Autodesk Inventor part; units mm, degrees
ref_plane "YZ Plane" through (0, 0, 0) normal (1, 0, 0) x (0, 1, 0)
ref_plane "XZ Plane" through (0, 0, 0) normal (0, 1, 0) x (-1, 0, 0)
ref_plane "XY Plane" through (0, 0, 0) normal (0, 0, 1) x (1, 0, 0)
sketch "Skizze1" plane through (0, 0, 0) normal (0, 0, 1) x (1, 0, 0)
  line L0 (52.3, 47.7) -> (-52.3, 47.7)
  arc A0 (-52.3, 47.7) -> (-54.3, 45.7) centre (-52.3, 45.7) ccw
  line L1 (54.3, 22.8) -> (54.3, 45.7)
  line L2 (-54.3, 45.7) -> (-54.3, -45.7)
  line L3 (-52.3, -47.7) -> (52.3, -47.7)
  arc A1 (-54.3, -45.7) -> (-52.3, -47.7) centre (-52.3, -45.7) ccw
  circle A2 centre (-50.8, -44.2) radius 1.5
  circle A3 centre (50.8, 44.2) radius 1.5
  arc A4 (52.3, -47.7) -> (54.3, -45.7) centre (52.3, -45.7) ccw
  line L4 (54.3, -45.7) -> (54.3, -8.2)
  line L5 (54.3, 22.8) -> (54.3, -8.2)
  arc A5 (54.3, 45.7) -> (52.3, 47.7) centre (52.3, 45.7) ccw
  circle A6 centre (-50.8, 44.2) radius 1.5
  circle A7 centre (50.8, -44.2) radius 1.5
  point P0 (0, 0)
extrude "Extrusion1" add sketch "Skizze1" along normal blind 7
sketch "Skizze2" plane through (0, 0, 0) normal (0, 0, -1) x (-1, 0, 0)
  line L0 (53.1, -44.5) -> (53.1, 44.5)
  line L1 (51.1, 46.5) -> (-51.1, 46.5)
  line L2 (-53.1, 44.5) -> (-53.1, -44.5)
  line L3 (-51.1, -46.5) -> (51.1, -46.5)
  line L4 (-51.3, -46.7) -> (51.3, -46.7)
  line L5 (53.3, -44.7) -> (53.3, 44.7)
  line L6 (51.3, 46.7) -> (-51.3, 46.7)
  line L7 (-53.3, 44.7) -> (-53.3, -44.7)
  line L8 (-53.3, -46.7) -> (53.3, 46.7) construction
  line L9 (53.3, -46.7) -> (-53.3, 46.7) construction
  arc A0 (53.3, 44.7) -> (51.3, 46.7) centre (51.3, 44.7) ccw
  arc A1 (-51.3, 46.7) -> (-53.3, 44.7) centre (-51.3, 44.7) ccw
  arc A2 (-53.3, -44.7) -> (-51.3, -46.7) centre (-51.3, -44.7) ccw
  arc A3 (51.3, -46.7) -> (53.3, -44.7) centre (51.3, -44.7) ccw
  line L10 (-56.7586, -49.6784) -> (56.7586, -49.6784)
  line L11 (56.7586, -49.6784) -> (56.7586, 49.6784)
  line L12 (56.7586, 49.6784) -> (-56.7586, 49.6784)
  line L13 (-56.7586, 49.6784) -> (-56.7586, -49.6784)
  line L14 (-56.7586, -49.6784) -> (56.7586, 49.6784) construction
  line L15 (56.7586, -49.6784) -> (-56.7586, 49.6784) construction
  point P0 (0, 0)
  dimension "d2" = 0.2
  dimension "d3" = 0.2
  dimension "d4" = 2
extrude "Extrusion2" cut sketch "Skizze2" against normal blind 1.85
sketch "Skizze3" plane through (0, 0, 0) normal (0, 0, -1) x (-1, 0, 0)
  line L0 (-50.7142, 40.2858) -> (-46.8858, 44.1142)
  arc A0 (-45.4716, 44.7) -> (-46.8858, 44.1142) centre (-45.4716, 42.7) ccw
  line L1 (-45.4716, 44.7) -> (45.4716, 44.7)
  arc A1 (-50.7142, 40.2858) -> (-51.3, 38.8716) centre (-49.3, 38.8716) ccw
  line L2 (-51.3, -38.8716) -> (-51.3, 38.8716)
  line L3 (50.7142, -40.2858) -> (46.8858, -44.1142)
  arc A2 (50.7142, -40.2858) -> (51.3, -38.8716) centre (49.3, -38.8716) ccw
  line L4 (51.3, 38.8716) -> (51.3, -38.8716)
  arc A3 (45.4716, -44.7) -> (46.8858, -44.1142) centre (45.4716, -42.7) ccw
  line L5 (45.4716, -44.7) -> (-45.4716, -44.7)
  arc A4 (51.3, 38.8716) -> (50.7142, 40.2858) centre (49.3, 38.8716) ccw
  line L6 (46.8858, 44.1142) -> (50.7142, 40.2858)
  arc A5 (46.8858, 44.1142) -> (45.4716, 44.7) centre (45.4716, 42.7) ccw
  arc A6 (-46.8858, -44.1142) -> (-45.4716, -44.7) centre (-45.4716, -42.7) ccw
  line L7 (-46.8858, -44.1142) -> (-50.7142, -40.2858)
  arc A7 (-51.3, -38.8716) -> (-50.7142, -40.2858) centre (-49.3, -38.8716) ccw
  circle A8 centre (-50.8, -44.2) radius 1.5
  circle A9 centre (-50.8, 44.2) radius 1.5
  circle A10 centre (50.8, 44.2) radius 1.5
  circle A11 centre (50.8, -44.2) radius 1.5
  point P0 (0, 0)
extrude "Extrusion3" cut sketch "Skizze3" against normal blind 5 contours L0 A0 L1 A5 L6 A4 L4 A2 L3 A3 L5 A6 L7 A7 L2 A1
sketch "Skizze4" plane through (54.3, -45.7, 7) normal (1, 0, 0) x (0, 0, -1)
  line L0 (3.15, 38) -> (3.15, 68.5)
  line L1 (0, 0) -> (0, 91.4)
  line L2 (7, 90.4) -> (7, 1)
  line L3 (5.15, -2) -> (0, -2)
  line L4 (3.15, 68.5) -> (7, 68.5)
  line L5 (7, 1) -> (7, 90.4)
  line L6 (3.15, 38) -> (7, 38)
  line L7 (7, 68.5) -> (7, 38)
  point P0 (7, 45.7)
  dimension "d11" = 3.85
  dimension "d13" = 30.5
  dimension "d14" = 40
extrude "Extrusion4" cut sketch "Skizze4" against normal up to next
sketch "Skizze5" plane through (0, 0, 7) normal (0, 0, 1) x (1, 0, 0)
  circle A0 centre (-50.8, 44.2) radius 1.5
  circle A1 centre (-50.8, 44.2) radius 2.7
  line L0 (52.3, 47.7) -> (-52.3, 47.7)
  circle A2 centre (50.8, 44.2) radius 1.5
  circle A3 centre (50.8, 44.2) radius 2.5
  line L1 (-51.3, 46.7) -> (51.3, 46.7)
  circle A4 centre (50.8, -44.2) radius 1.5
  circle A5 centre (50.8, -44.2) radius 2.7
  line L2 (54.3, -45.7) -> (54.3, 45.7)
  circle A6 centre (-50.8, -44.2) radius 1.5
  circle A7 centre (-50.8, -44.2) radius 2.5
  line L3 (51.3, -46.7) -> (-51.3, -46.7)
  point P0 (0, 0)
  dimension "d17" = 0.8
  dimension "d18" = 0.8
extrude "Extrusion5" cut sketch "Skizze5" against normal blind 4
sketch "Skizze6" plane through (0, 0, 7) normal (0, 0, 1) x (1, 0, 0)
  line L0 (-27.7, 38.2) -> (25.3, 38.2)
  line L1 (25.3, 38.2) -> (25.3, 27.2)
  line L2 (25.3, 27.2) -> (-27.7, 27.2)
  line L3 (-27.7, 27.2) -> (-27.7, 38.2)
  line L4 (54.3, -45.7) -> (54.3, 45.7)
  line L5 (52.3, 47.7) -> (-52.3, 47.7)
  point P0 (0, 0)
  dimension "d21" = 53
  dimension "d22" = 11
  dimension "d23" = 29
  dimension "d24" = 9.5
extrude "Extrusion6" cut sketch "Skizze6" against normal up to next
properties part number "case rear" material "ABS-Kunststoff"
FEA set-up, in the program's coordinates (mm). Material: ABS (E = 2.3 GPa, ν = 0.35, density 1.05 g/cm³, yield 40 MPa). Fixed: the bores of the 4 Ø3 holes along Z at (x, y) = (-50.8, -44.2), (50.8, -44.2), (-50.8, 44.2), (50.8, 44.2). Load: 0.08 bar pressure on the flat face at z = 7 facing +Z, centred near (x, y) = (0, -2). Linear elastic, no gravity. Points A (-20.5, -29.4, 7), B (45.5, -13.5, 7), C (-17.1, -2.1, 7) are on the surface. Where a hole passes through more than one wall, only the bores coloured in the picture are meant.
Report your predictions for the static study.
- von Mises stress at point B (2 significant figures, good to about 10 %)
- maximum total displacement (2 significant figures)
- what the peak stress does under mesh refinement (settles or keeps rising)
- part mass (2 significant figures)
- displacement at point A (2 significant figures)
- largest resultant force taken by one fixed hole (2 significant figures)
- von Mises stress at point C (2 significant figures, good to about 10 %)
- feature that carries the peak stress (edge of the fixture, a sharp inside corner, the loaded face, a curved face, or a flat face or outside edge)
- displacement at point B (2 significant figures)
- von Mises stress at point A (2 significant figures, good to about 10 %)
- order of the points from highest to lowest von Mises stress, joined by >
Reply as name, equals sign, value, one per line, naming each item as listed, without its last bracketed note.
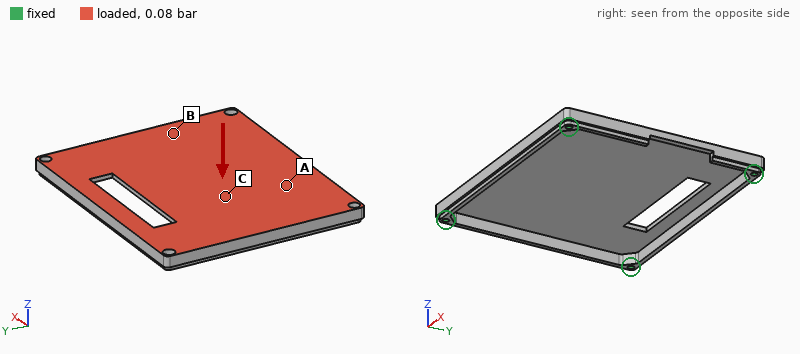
von Mises stress at point B = 1.7 MPa
maximum total displacement = 1.7 mm
what the peak stress does under mesh refinement = keeps rising
part mass = 25 g
displacement at point A = 0.78 mm
largest resultant force taken by one fixed hole = 63 N
von Mises stress at point C = 4.4 MPa
feature that carries the peak stress = edge of the fixture
displacement at point B = 0.45 mm
von Mises stress at point A = 2.8 MPa
order of the points from highest to lowest von Mises stress, joined by > = C > A > B
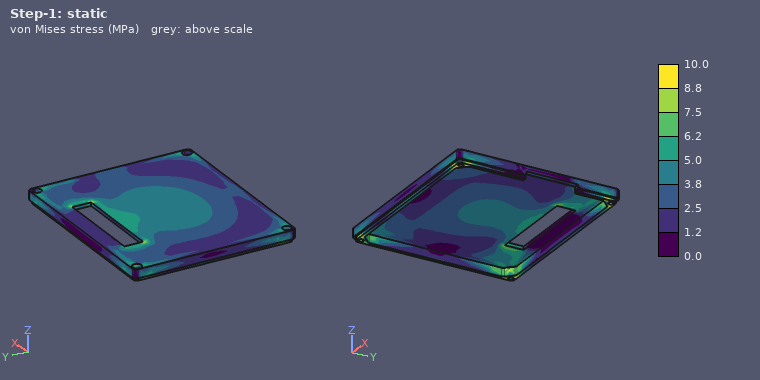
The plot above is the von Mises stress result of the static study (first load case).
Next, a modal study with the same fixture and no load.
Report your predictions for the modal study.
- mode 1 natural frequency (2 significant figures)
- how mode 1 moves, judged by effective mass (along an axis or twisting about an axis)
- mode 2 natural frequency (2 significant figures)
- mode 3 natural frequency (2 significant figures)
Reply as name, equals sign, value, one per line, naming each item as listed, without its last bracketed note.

mode 1 natural frequency = 290 Hz
how mode 1 moves, judged by effective mass = along Z
mode 2 natural frequency = 600 Hz
mode 3 natural frequency = 620 Hz
